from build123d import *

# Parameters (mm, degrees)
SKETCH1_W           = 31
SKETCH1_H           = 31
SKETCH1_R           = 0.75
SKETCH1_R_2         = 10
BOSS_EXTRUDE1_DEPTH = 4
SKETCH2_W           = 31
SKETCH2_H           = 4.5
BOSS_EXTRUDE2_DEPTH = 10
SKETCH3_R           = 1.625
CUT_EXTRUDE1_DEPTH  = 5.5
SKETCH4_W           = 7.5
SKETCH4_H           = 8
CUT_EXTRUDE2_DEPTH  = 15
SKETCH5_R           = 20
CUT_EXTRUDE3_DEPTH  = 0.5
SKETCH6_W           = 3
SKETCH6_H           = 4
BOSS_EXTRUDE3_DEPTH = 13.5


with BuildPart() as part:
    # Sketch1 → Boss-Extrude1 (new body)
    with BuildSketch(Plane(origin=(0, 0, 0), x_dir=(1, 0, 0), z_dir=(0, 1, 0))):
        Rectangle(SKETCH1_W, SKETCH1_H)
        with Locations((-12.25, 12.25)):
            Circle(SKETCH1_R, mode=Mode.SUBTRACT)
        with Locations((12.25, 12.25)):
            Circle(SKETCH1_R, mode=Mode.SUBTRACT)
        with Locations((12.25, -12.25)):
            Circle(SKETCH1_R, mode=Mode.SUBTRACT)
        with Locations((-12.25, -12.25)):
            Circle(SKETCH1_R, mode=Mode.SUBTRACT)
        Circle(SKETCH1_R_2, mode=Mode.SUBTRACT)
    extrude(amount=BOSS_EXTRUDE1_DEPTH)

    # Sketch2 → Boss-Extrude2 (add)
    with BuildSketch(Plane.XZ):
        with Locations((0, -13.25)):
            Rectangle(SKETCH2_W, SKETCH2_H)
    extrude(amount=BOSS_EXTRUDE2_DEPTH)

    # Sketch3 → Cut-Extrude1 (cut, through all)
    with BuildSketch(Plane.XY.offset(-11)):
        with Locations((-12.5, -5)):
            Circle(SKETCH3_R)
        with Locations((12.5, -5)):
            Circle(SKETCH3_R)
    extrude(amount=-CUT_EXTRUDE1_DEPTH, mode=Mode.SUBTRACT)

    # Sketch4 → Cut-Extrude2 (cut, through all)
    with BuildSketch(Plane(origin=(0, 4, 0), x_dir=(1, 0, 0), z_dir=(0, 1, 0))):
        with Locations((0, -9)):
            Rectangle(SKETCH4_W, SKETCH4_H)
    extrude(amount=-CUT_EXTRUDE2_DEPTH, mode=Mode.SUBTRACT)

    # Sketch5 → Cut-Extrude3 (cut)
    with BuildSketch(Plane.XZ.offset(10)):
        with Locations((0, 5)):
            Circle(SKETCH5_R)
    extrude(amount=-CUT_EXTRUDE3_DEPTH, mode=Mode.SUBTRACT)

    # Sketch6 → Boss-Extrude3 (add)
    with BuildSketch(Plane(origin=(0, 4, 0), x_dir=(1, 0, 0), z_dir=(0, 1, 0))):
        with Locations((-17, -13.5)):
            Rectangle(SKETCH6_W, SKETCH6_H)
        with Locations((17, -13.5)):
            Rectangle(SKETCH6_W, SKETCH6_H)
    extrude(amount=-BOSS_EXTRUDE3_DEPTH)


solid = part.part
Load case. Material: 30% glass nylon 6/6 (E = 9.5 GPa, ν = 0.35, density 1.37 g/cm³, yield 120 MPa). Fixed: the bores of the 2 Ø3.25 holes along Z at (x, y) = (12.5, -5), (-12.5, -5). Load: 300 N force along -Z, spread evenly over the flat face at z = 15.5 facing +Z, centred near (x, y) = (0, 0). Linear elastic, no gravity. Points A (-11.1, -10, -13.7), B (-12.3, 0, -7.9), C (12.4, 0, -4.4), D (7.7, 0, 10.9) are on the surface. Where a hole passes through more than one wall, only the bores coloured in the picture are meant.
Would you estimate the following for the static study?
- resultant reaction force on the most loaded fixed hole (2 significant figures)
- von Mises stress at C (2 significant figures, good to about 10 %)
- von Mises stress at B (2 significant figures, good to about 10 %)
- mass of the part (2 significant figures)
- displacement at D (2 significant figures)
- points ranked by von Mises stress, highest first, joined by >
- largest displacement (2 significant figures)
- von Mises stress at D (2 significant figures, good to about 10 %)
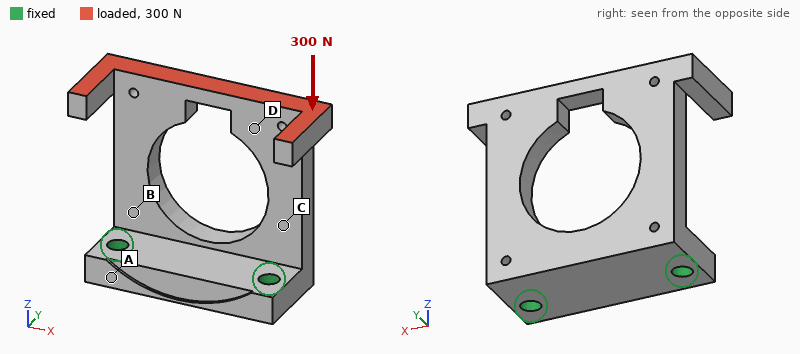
150 N
23 MPa
19 MPa
5.6 g
0.17 mm
C > B > D > A
0.43 mm
6.5 MPa
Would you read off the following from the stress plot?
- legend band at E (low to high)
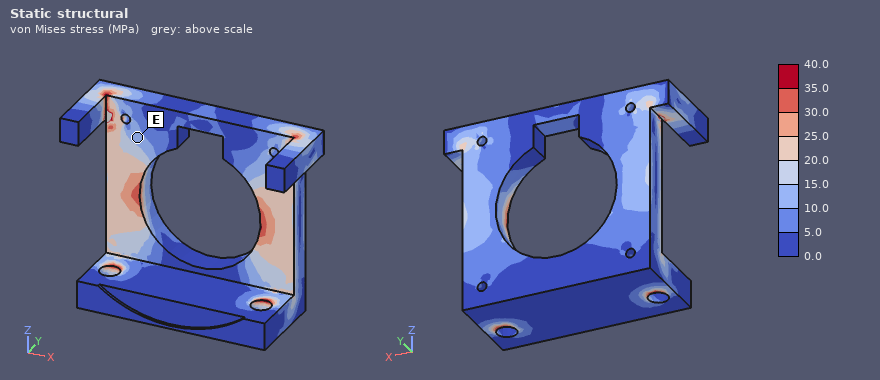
10.0 to 15.0 MPa
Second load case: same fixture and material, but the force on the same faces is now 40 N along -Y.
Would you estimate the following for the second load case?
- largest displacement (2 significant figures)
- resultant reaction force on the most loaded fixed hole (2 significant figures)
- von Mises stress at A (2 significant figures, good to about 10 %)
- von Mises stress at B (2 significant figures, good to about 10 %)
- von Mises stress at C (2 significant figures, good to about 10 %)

0.59 mm
21 N
3.3 MPa
21 MPa
23 MPa
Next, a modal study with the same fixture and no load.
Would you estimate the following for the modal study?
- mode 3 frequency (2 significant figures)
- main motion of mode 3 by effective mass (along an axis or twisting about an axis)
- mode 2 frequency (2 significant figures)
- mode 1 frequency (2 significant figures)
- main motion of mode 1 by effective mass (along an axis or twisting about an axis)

3400 Hz
along X
2100 Hz
1200 Hz
along Y
